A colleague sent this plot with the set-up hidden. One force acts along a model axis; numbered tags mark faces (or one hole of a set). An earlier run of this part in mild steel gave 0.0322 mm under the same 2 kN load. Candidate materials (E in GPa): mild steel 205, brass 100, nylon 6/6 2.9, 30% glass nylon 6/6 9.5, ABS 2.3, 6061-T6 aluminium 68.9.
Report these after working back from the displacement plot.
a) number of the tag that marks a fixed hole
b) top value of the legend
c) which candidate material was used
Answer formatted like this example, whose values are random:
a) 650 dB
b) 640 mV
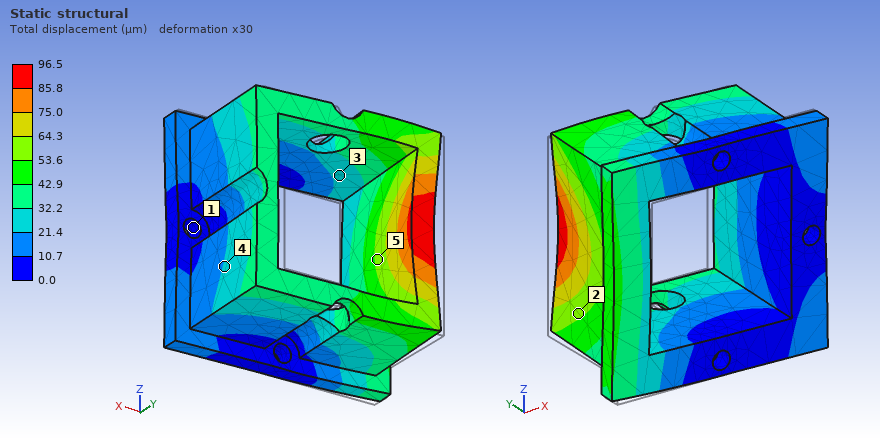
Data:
a) 1
b) 96.5 µm
c) 6061-T6 aluminium
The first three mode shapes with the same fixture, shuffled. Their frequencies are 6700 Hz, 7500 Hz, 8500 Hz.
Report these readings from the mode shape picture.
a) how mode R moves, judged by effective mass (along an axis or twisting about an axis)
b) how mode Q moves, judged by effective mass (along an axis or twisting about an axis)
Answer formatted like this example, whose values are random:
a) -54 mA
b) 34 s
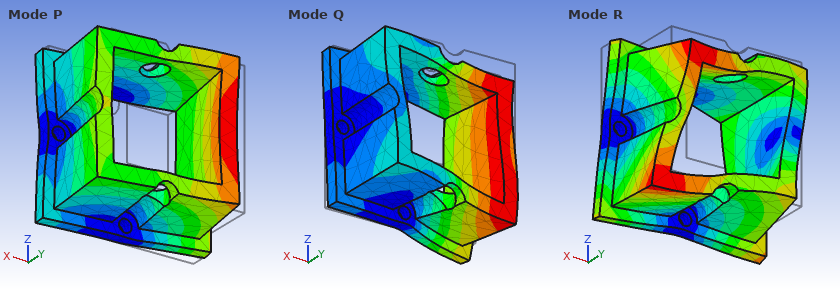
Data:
a) along Z
b) along Z
